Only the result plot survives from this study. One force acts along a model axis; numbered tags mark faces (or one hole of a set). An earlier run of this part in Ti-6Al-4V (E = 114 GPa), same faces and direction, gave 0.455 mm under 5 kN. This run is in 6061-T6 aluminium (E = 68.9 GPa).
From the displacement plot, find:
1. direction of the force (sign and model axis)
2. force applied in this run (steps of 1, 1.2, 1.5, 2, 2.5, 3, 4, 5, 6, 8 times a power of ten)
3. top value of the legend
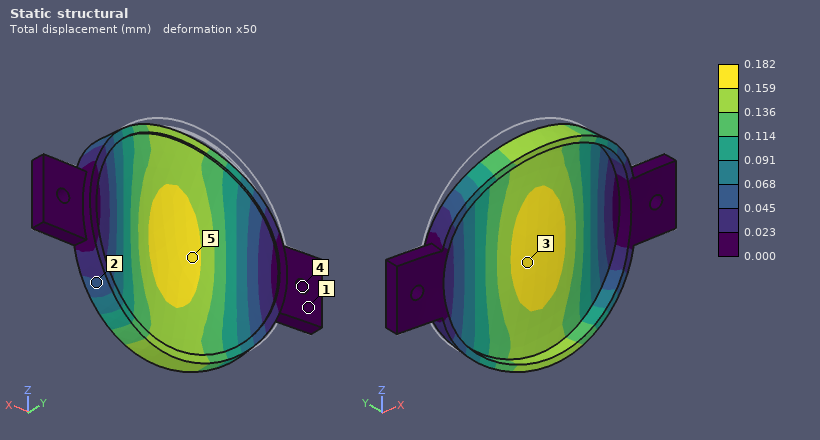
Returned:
-Y
1.2 kN
0.182 mm
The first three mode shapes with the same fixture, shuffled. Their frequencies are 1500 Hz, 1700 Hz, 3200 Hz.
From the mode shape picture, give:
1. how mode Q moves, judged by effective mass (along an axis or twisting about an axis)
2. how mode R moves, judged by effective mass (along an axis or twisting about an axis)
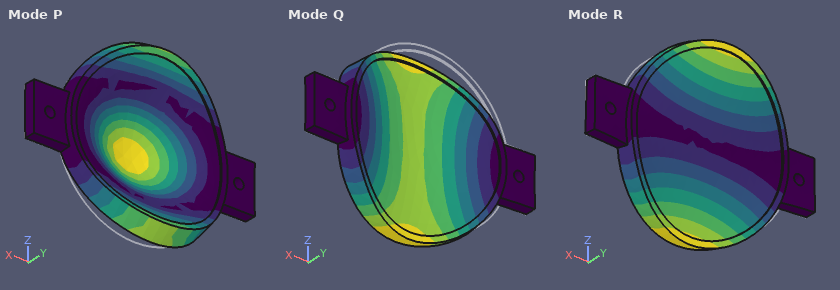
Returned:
along Y
twisting about X
